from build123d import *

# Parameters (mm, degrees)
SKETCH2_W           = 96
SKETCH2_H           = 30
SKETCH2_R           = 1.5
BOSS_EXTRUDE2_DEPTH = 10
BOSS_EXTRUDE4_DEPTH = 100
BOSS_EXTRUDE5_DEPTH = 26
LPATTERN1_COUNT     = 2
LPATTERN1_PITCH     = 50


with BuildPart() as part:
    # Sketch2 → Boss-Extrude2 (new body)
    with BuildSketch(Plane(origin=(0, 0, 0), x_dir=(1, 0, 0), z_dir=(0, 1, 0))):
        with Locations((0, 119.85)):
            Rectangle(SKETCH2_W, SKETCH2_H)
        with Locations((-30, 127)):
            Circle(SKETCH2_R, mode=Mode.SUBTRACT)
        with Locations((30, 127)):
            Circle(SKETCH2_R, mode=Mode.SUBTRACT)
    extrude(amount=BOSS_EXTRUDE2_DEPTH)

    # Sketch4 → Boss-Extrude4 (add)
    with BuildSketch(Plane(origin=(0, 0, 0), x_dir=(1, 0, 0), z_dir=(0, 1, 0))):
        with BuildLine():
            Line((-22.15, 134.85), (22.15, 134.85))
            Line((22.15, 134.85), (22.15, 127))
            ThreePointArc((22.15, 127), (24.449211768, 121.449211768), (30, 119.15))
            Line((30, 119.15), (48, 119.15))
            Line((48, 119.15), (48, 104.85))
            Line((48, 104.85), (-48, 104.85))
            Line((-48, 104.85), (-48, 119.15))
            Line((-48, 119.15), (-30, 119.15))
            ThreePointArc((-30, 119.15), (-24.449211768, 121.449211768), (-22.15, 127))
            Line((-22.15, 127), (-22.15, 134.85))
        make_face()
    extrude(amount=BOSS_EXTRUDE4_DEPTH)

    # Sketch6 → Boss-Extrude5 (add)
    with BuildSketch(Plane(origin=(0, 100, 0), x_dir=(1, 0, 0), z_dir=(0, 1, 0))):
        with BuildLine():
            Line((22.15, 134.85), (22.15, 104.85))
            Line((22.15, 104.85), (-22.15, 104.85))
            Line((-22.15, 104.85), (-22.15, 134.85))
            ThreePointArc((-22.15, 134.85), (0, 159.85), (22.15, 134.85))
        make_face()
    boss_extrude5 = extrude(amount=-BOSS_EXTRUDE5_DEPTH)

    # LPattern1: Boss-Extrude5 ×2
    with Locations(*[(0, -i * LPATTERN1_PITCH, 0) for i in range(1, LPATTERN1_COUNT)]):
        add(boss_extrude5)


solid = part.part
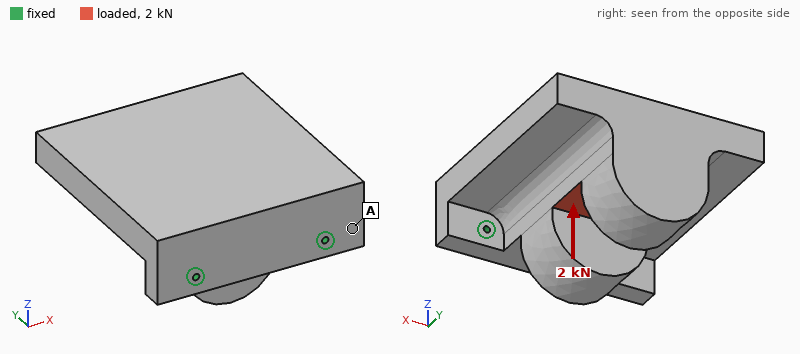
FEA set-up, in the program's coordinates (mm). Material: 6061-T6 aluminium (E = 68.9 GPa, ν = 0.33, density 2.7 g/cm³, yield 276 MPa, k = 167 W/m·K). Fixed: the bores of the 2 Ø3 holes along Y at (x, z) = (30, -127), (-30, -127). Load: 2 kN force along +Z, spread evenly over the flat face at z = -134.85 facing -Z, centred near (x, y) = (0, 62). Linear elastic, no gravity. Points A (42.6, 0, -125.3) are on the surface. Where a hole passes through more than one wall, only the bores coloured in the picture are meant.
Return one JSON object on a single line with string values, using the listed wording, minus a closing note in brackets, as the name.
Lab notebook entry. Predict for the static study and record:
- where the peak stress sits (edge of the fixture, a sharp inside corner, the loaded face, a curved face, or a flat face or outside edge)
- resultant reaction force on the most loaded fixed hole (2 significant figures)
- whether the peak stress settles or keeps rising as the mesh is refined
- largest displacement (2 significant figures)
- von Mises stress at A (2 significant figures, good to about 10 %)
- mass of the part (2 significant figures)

{"where the peak stress sits": "edge of the fixture", "resultant reaction force on the most loaded fixed hole": "1.3 kN", "whether the peak stress settles or keeps rising as the mesh is refined": "keeps rising", "largest displacement": "0.47 mm", "von Mises stress at A": "30 MPa", "mass of the part": "710 g"}
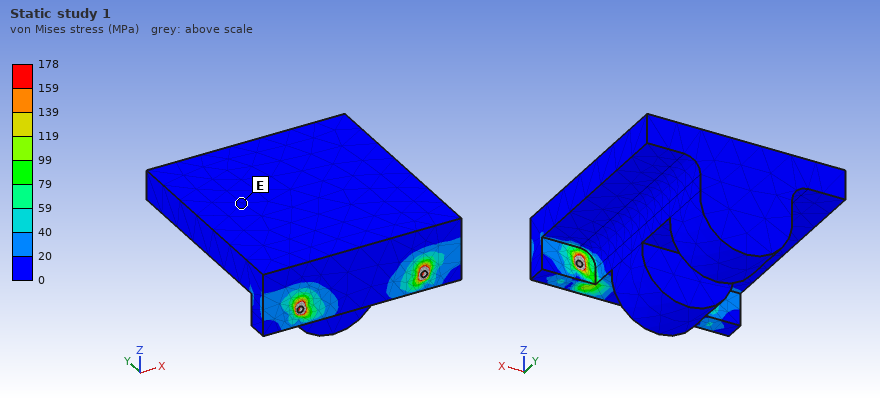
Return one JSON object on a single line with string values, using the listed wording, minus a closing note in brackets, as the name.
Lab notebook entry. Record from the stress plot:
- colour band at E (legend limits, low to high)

{"colour band at E": "0 to 20 MPa"}
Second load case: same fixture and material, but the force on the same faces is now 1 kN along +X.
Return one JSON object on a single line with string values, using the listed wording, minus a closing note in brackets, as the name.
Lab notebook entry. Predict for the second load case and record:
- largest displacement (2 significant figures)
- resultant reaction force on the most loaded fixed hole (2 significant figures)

{"largest displacement": "18 µm", "resultant reaction force on the most loaded fixed hole": "1.1 kN"}
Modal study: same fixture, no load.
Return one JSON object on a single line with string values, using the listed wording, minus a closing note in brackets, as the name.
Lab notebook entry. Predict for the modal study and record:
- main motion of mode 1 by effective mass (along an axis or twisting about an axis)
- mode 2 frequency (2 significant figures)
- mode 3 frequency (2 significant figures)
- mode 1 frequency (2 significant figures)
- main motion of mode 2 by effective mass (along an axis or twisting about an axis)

{"main motion of mode 1 by effective mass": "along Z", "mode 2 frequency": "2000 Hz", "mode 3 frequency": "3700 Hz", "mode 1 frequency": "530 Hz", "main motion of mode 2 by effective mass": "along X"}
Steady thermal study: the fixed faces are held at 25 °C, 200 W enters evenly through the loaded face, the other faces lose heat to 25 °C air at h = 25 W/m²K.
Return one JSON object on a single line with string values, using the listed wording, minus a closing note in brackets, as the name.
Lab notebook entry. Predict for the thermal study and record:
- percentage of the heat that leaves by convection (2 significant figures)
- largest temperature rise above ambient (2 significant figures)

{"percentage of the heat that leaves by convection": "17 %", "largest temperature rise above ambient": "60 K"}
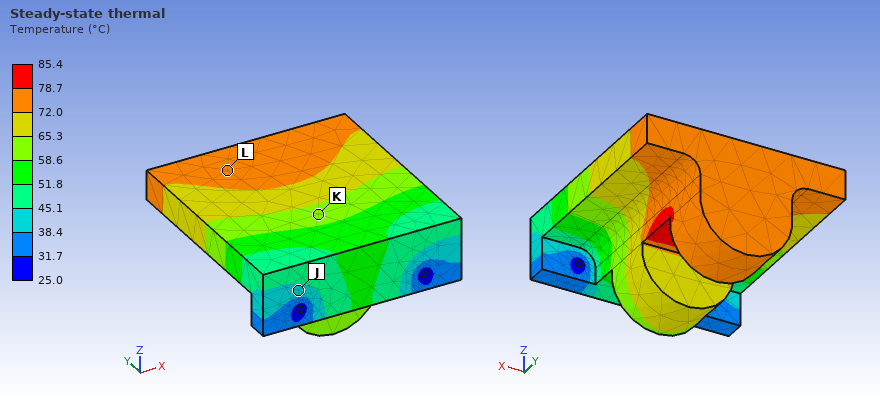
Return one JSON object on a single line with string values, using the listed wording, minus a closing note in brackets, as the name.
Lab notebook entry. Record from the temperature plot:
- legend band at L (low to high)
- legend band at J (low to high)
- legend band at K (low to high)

{"legend band at L": "72.0 to 78.7 °C", "legend band at J": "38.4 to 45.1 °C", "legend band at K": "58.6 to 65.3 °C"}
